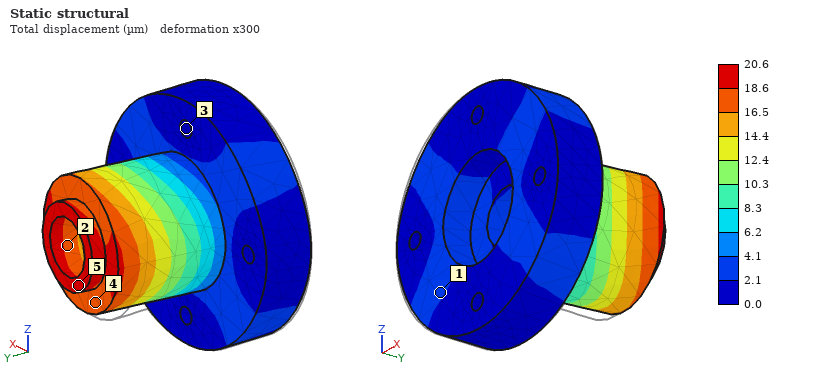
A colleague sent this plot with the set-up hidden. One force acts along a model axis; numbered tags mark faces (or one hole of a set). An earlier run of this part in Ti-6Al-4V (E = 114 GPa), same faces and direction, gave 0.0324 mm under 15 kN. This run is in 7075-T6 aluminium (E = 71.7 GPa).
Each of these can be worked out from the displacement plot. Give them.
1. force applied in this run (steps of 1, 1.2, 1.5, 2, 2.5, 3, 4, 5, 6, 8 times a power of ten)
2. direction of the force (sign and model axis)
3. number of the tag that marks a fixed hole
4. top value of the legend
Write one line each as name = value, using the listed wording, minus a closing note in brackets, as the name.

force applied in this run = 6 kN
direction of the force = +X
number of the tag that marks a fixed hole = 3
top value of the legend = 20.6 µm
